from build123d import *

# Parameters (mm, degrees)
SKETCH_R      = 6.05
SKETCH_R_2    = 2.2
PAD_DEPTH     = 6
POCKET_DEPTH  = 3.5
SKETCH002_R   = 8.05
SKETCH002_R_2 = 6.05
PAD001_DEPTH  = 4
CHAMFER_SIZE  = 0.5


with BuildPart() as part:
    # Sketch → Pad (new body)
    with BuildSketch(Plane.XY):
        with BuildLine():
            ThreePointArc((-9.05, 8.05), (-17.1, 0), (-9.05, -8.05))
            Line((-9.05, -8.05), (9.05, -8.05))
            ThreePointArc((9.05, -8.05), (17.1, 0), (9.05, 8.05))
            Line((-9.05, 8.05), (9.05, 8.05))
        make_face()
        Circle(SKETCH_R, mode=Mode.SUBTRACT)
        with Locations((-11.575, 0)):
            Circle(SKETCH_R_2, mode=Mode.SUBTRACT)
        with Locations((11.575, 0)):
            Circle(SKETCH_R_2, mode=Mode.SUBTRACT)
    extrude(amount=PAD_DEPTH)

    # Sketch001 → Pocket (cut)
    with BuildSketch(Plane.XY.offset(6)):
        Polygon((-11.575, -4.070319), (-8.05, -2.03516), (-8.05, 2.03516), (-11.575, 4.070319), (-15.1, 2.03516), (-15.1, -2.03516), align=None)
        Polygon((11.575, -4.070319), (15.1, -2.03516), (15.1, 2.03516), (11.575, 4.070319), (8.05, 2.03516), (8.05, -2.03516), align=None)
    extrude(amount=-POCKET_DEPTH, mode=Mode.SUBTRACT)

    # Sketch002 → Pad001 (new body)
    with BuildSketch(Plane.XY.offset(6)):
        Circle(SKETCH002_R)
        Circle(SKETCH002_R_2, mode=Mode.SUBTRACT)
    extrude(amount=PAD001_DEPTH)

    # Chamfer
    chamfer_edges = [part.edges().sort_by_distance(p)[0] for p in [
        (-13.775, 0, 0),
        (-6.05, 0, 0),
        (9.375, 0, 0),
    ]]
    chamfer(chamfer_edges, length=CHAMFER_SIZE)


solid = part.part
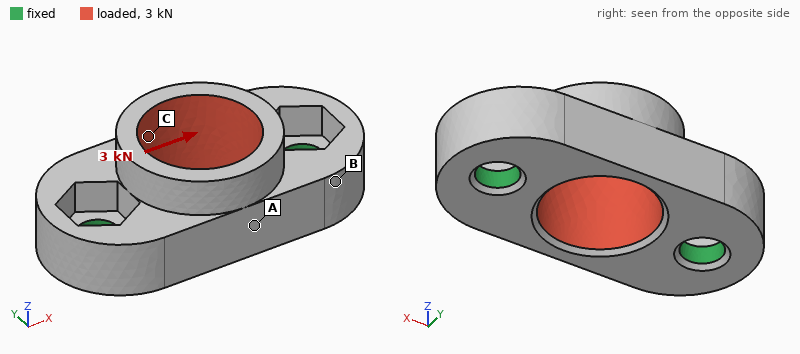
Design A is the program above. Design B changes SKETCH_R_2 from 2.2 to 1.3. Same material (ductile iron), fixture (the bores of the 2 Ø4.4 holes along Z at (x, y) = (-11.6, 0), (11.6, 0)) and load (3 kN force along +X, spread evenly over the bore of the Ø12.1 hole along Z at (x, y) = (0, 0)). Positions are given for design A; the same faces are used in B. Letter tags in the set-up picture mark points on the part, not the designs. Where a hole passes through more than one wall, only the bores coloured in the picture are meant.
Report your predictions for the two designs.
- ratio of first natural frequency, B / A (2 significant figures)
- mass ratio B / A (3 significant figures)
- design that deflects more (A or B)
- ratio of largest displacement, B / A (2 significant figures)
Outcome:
0.70
1.02
B
1.2
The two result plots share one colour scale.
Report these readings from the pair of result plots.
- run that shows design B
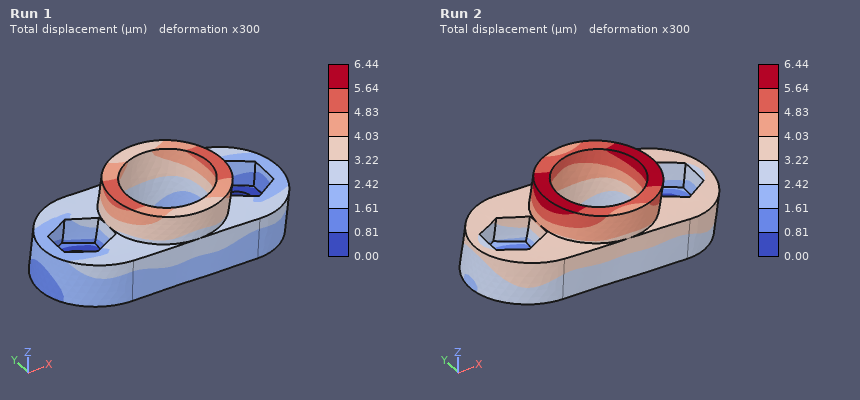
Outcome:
Run 2
